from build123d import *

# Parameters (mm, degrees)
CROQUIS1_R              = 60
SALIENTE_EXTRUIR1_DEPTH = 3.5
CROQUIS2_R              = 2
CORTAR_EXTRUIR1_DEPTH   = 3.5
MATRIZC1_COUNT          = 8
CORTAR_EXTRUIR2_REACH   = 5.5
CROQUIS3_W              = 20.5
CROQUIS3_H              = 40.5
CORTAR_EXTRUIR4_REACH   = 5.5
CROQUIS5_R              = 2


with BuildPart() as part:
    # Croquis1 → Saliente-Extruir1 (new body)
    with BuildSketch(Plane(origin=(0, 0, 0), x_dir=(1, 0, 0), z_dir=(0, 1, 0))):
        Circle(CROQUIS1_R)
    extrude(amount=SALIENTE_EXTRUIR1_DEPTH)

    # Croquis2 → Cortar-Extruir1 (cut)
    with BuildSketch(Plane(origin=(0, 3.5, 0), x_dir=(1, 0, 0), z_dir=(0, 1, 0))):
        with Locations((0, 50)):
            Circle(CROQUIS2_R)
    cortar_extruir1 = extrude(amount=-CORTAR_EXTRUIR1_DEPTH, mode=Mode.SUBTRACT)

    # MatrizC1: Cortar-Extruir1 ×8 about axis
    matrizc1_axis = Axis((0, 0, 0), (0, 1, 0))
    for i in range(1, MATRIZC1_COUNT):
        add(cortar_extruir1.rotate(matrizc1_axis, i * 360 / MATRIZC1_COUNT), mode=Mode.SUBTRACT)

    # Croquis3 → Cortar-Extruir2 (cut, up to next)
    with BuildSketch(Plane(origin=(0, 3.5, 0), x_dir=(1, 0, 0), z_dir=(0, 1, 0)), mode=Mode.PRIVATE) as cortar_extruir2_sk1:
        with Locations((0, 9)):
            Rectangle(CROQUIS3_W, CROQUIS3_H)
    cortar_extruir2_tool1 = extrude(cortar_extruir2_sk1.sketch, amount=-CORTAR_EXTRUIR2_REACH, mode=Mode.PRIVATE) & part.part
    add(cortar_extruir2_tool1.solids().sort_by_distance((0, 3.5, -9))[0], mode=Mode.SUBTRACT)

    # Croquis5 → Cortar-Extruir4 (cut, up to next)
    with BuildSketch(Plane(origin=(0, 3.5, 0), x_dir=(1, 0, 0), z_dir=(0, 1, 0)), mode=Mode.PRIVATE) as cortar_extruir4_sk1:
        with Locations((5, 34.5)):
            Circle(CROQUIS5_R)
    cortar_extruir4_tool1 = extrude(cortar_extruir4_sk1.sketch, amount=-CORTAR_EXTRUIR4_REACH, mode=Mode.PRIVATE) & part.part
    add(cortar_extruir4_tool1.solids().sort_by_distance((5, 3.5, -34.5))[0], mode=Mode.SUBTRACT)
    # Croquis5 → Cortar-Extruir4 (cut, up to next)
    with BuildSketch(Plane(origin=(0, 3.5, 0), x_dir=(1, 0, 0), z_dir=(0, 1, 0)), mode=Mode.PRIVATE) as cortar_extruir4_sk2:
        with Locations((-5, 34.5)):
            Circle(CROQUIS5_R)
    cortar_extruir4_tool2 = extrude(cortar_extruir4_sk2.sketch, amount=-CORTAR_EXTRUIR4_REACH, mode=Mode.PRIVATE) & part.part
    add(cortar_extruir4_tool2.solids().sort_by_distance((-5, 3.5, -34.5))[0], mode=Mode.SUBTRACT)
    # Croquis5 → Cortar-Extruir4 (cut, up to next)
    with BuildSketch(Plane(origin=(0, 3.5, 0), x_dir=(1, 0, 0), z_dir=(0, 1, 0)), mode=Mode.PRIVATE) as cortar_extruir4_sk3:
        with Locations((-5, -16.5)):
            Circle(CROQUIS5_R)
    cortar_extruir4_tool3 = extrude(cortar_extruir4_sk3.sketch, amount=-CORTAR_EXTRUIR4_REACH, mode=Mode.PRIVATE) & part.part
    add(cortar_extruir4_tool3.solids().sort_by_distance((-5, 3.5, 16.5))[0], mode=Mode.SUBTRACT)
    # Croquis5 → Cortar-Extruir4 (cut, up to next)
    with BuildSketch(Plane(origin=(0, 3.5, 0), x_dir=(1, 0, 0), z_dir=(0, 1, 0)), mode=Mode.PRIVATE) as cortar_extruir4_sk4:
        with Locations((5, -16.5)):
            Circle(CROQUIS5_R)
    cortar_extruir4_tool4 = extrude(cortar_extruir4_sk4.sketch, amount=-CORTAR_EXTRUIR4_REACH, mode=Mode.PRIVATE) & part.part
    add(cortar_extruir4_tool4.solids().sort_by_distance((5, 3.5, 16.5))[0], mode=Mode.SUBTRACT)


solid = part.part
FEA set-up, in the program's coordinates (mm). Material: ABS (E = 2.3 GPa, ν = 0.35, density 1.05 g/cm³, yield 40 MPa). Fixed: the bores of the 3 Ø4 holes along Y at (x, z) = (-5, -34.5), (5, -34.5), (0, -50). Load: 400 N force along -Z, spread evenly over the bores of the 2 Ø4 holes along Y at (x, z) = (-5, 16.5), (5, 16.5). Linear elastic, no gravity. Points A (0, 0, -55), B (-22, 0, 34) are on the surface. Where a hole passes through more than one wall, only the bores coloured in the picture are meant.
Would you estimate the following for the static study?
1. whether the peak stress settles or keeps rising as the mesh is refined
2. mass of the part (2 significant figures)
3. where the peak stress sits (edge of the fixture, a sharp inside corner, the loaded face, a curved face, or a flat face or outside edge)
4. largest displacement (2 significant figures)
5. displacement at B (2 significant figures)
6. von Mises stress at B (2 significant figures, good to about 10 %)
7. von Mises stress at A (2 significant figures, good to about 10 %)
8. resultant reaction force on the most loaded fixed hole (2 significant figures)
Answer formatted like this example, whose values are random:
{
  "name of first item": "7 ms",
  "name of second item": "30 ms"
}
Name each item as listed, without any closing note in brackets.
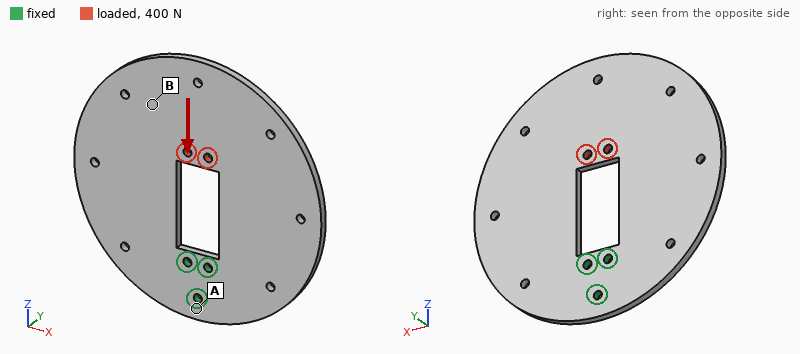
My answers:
{
  "whether the peak stress settles or keeps rising as the mesh is refined": "keeps rising",
  "mass of the part": "38 g",
  "where the peak stress sits": "edge of the fixture",
  "largest displacement": "0.16 mm",
  "displacement at B": "0.11 mm",
  "von Mises stress at B": "1.4 MPa",
  "von Mises stress at A": "3.2 MPa",
  "resultant reaction force on the most loaded fixed hole": "160 N"
}
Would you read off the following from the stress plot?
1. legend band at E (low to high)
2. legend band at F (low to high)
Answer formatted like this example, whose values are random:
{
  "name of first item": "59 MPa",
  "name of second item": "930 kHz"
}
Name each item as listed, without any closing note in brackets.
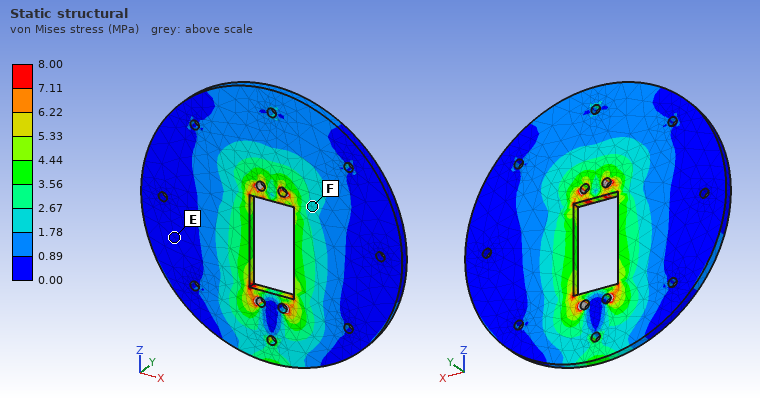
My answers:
{
  "legend band at E": "0.00 to 0.89 MPa",
  "legend band at F": "1.78 to 2.67 MPa"
}
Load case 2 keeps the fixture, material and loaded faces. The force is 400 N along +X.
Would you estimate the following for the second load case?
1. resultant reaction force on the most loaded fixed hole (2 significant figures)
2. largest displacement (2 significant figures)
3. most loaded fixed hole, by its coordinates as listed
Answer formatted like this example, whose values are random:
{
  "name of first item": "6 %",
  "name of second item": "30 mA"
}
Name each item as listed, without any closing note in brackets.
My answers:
{
  "resultant reaction force on the most loaded fixed hole": "980 N",
  "largest displacement": "1.6 mm",
  "most loaded fixed hole, by its coordinates as listed": "(0, -50)"
}
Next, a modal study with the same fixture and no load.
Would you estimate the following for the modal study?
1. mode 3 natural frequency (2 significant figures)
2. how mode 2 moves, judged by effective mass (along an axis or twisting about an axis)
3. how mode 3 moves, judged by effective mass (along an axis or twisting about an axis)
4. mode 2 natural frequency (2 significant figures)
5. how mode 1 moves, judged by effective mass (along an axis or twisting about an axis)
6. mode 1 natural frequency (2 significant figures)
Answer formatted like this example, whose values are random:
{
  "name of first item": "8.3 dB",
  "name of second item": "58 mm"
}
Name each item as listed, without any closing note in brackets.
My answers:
{
  "mode 3 natural frequency": "290 Hz",
  "how mode 2 moves, judged by effective mass": "twisting about Z",
  "how mode 3 moves, judged by effective mass": "along Y",
  "mode 2 natural frequency": "130 Hz",
  "how mode 1 moves, judged by effective mass": "along Y",
  "mode 1 natural frequency": "75 Hz"
}
